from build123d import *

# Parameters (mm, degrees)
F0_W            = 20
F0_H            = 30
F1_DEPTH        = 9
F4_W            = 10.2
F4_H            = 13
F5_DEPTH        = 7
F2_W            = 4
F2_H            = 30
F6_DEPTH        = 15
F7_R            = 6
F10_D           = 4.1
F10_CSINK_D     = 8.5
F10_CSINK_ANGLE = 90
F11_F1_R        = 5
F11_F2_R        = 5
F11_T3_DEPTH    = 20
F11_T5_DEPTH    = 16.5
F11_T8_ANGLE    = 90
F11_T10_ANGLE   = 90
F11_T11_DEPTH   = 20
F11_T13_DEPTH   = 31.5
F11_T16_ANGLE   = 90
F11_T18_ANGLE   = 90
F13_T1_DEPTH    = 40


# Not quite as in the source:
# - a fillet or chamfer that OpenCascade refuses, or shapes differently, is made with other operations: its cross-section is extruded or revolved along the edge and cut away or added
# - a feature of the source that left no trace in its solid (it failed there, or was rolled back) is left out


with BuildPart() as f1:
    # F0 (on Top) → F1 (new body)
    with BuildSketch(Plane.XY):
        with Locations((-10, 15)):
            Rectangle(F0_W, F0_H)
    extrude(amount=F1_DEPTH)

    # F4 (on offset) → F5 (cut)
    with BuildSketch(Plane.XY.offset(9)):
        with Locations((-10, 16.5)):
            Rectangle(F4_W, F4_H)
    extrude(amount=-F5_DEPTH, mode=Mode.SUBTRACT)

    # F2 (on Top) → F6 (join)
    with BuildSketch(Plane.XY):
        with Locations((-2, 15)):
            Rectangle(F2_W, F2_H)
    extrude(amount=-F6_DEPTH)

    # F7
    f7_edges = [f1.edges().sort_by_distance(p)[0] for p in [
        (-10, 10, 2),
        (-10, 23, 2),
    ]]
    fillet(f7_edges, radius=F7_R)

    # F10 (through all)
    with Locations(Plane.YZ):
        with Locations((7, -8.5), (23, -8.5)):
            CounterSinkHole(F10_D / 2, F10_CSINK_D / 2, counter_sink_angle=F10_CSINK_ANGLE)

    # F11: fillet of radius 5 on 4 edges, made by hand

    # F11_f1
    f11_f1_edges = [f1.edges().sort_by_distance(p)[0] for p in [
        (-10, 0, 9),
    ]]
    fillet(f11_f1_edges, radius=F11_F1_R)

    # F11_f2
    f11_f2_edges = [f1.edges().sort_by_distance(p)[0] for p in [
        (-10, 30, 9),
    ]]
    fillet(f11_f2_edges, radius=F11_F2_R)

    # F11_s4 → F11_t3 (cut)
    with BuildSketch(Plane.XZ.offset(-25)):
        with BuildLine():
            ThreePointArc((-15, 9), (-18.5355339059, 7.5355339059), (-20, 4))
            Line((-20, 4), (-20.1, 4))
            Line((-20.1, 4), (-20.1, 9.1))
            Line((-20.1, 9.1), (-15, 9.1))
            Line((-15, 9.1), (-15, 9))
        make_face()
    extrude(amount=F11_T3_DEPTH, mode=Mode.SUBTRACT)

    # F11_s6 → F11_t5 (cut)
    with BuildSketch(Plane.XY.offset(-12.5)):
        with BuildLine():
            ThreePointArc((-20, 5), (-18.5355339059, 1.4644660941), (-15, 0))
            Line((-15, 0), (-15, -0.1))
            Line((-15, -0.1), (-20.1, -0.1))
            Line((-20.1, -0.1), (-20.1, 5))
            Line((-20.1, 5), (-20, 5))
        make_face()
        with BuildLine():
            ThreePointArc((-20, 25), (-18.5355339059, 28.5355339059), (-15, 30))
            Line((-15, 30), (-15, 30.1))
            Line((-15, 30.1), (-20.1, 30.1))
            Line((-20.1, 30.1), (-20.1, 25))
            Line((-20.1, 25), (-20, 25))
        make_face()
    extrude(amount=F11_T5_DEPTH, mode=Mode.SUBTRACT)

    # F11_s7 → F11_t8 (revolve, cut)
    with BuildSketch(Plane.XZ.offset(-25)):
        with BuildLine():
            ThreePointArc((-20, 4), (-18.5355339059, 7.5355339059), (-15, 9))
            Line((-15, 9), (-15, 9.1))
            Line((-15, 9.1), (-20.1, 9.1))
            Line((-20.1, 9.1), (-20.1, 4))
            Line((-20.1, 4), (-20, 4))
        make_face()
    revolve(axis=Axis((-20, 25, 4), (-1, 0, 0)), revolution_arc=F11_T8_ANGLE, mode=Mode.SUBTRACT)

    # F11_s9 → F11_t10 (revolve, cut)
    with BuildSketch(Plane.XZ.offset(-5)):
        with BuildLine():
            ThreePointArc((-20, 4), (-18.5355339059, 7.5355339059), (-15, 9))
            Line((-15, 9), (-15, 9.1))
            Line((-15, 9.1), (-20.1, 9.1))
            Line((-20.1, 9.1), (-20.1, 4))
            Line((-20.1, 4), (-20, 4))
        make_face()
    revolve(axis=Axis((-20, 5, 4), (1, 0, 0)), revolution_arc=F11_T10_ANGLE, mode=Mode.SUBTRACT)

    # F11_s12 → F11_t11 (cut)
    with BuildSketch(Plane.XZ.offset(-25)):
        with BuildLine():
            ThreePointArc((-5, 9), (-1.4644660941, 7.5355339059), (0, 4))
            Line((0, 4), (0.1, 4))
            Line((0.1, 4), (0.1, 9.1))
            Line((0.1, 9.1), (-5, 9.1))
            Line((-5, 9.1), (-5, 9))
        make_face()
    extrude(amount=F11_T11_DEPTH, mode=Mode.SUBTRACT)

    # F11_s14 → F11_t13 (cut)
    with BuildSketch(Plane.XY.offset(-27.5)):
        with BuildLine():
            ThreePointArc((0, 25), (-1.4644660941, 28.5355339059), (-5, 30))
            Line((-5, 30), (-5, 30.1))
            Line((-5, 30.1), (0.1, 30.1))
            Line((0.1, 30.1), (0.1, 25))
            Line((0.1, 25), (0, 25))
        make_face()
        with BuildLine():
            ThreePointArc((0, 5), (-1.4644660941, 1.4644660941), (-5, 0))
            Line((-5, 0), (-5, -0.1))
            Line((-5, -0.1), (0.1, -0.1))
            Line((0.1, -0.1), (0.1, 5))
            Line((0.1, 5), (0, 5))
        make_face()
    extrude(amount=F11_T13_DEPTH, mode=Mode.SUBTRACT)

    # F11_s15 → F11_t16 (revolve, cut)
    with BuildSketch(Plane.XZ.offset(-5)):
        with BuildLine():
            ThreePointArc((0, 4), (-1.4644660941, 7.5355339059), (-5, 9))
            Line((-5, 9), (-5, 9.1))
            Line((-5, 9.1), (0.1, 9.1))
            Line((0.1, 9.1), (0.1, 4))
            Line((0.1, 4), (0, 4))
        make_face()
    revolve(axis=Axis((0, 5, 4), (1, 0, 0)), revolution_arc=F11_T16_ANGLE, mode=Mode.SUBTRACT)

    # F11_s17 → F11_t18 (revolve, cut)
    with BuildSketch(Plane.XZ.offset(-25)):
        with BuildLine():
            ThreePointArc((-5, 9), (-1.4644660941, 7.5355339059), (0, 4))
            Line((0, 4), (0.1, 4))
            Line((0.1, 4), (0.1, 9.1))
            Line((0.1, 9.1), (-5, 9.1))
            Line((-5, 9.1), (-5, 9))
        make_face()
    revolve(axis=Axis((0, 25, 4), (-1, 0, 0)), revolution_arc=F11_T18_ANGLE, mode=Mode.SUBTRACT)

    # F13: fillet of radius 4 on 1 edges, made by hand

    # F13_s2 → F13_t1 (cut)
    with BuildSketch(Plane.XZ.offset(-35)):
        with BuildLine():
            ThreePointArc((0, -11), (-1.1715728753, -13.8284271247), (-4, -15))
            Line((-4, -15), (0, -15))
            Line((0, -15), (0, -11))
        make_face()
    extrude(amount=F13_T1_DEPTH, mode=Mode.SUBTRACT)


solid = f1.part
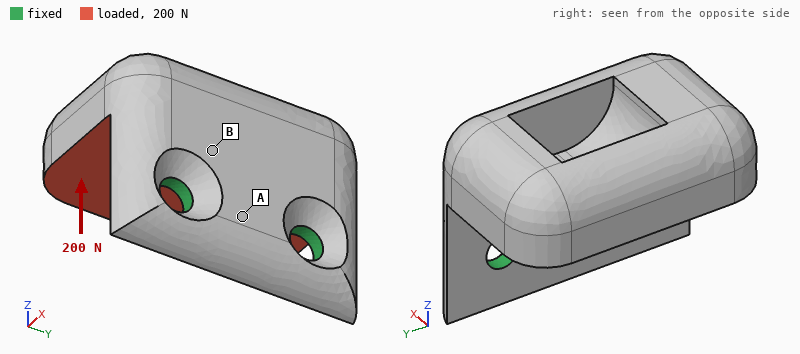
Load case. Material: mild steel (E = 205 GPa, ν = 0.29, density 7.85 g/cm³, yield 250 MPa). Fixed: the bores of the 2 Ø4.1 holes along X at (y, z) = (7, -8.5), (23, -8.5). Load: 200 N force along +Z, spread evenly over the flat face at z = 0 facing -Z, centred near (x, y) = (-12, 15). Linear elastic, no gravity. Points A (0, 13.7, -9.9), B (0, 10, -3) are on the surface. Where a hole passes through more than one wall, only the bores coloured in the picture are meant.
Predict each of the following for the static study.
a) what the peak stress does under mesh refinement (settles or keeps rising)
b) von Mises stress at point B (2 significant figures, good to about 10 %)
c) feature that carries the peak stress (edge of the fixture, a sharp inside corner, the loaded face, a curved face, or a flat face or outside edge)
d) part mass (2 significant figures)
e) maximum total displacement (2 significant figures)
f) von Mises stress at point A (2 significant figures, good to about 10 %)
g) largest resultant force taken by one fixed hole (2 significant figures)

keeps rising
25 MPa
edge of the fixture
42 g
20 µm
9.7 MPa
100 N
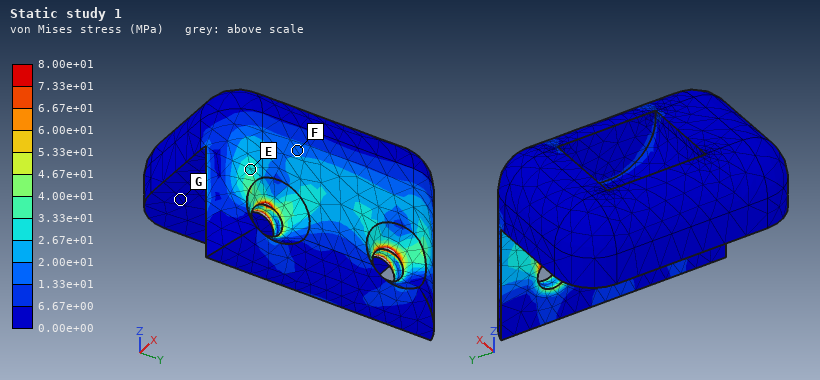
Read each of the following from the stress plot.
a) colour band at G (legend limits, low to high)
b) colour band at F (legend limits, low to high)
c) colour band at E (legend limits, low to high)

0.00e+00 to 6.67e+00 MPa
1.33e+01 to 2.00e+01 MPa
2.67e+01 to 3.33e+01 MPa
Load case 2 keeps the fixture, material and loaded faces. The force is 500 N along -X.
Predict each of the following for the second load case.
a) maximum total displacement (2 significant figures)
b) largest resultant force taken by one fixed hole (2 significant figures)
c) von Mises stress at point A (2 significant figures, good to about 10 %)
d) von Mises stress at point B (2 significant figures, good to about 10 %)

24 µm
250 N
18 MPa
26 MPa
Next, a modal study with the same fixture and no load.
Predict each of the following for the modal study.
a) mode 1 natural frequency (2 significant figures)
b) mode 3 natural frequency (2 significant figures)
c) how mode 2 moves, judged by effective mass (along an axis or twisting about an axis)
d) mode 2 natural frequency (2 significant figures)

3000 Hz
13 kHz
along Y
6700 Hz
